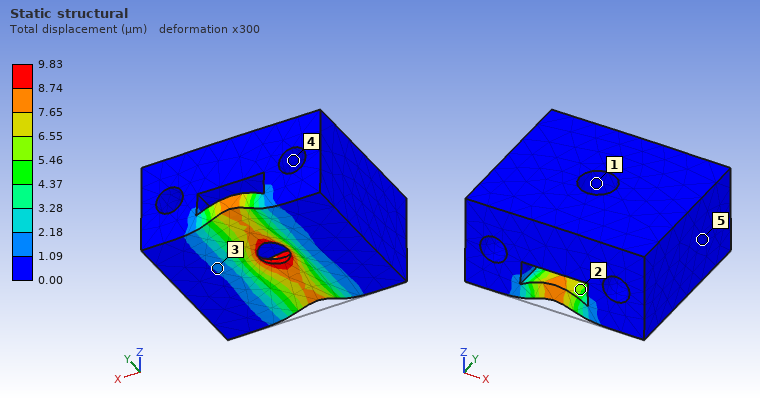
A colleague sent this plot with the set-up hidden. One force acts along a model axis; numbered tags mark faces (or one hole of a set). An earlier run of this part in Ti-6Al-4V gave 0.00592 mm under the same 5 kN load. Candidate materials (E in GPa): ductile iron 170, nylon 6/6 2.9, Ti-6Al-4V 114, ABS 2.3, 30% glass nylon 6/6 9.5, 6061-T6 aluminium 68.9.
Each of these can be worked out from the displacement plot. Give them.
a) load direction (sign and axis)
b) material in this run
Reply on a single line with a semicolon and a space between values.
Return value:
+Z; 6061-T6 aluminium
